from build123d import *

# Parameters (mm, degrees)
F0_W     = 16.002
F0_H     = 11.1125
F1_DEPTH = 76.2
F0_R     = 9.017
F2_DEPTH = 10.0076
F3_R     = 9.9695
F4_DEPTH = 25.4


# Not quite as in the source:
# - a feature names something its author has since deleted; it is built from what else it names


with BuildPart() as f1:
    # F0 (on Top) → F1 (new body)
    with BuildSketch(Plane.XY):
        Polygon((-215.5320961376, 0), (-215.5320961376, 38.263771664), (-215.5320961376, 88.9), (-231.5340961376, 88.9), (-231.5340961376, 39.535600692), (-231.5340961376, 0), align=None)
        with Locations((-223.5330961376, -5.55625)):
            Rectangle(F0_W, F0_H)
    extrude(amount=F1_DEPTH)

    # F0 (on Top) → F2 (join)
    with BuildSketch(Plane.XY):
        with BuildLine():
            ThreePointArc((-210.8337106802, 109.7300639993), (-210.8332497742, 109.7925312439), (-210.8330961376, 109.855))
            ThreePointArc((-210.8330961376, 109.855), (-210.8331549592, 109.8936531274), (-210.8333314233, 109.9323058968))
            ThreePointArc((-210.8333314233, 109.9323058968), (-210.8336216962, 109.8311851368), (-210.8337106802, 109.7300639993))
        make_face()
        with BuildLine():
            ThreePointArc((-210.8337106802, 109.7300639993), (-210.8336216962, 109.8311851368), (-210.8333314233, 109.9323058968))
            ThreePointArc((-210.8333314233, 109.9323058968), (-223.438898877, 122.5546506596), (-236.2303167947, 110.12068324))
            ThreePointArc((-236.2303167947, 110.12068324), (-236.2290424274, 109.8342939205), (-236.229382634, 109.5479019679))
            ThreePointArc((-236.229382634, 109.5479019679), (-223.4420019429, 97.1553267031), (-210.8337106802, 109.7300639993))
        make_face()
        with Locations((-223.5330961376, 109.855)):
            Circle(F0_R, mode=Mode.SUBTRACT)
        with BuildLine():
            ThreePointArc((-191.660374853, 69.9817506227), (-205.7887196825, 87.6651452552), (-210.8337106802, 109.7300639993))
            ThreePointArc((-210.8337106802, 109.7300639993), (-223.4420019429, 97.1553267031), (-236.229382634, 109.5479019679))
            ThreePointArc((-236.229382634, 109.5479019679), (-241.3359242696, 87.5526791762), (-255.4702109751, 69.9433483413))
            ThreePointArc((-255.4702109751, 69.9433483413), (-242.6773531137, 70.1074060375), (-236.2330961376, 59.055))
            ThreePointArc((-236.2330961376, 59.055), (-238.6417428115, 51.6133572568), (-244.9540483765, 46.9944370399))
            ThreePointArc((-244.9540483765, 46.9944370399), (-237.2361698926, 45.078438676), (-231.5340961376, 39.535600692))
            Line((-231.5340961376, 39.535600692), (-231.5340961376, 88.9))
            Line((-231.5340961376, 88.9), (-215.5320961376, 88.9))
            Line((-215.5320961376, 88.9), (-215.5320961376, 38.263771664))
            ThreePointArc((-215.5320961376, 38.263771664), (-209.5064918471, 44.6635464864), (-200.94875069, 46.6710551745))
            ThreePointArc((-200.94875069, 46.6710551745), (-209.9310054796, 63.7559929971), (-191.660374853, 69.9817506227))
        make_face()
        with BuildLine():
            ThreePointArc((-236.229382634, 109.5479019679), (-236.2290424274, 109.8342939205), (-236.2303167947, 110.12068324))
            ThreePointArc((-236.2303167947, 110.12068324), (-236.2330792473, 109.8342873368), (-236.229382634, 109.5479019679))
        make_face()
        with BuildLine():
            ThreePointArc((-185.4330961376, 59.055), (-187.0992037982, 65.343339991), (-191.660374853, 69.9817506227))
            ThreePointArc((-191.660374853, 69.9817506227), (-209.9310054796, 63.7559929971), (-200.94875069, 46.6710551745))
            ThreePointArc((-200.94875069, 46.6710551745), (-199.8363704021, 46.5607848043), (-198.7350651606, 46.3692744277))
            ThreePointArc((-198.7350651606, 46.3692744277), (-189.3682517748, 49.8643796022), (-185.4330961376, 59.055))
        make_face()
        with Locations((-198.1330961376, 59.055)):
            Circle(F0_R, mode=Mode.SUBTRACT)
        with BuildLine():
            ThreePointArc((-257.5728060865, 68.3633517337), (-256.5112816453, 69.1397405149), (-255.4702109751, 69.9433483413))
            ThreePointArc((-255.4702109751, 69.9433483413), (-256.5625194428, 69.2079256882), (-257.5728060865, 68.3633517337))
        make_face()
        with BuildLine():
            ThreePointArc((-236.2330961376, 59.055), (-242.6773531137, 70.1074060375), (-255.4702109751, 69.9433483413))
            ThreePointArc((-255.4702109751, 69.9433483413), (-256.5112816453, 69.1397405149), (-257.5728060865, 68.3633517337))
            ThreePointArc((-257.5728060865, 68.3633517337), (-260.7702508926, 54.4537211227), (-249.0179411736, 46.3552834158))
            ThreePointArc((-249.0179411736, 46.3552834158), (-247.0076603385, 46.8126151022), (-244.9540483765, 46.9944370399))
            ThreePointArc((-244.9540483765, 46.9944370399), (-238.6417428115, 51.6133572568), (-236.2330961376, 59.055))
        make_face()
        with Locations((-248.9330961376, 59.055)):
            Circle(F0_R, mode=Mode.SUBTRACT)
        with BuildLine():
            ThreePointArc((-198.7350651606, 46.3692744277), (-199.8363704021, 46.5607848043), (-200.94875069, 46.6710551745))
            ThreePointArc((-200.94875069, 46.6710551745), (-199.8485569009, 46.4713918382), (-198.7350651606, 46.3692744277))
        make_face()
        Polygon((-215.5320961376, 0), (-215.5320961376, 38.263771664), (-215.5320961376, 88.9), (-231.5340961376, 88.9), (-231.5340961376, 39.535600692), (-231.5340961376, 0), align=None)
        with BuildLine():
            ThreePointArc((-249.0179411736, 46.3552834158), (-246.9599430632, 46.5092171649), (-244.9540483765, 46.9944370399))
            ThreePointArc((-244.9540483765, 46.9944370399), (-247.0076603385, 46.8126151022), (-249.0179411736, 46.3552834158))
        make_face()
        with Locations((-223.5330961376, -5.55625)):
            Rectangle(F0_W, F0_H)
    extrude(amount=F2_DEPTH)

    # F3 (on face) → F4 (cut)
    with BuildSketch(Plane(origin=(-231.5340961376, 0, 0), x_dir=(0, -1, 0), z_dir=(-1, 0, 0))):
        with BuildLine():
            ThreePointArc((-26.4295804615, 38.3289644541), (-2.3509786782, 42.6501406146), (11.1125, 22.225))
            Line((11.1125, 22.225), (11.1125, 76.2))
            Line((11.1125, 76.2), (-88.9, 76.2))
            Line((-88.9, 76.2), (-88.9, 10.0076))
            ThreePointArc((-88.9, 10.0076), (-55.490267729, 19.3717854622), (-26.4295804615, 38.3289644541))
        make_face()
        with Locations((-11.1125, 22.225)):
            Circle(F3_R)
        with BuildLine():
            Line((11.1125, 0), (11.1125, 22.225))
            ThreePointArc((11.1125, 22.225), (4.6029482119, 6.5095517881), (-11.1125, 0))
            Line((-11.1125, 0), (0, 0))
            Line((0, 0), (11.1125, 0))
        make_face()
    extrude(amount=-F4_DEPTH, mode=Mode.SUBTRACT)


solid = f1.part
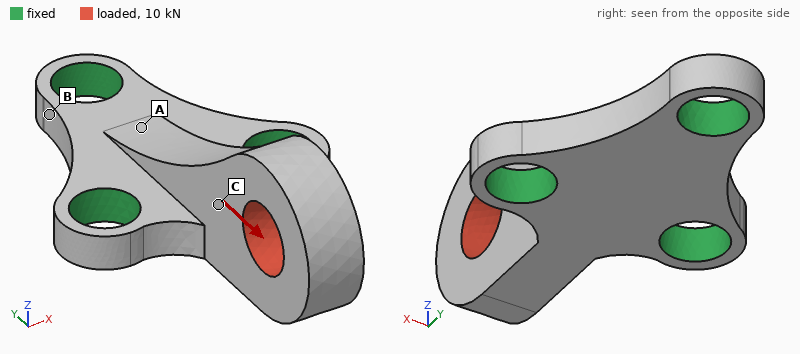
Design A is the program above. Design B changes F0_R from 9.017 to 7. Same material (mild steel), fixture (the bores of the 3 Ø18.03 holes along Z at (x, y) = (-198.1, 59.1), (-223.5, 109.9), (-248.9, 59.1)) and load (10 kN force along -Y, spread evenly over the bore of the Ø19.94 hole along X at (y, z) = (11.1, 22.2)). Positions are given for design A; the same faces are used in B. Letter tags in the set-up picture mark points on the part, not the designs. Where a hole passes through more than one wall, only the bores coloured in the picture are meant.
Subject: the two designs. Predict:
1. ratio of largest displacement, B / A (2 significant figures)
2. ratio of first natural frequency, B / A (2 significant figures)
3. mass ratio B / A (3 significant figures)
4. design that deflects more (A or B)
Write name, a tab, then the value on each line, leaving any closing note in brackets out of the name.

ratio of largest displacement, B / A	1.1
ratio of first natural frequency, B / A	0.94
mass ratio B / A	1.05
design that deflects more	B
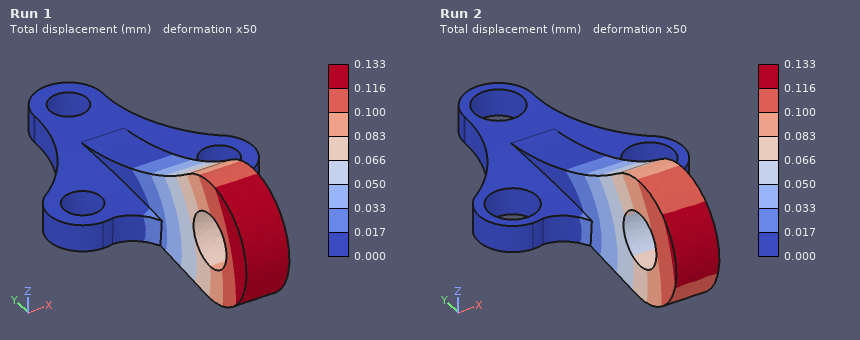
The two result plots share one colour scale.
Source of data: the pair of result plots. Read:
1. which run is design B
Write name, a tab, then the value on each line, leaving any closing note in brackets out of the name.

which run is design B	Run 1
